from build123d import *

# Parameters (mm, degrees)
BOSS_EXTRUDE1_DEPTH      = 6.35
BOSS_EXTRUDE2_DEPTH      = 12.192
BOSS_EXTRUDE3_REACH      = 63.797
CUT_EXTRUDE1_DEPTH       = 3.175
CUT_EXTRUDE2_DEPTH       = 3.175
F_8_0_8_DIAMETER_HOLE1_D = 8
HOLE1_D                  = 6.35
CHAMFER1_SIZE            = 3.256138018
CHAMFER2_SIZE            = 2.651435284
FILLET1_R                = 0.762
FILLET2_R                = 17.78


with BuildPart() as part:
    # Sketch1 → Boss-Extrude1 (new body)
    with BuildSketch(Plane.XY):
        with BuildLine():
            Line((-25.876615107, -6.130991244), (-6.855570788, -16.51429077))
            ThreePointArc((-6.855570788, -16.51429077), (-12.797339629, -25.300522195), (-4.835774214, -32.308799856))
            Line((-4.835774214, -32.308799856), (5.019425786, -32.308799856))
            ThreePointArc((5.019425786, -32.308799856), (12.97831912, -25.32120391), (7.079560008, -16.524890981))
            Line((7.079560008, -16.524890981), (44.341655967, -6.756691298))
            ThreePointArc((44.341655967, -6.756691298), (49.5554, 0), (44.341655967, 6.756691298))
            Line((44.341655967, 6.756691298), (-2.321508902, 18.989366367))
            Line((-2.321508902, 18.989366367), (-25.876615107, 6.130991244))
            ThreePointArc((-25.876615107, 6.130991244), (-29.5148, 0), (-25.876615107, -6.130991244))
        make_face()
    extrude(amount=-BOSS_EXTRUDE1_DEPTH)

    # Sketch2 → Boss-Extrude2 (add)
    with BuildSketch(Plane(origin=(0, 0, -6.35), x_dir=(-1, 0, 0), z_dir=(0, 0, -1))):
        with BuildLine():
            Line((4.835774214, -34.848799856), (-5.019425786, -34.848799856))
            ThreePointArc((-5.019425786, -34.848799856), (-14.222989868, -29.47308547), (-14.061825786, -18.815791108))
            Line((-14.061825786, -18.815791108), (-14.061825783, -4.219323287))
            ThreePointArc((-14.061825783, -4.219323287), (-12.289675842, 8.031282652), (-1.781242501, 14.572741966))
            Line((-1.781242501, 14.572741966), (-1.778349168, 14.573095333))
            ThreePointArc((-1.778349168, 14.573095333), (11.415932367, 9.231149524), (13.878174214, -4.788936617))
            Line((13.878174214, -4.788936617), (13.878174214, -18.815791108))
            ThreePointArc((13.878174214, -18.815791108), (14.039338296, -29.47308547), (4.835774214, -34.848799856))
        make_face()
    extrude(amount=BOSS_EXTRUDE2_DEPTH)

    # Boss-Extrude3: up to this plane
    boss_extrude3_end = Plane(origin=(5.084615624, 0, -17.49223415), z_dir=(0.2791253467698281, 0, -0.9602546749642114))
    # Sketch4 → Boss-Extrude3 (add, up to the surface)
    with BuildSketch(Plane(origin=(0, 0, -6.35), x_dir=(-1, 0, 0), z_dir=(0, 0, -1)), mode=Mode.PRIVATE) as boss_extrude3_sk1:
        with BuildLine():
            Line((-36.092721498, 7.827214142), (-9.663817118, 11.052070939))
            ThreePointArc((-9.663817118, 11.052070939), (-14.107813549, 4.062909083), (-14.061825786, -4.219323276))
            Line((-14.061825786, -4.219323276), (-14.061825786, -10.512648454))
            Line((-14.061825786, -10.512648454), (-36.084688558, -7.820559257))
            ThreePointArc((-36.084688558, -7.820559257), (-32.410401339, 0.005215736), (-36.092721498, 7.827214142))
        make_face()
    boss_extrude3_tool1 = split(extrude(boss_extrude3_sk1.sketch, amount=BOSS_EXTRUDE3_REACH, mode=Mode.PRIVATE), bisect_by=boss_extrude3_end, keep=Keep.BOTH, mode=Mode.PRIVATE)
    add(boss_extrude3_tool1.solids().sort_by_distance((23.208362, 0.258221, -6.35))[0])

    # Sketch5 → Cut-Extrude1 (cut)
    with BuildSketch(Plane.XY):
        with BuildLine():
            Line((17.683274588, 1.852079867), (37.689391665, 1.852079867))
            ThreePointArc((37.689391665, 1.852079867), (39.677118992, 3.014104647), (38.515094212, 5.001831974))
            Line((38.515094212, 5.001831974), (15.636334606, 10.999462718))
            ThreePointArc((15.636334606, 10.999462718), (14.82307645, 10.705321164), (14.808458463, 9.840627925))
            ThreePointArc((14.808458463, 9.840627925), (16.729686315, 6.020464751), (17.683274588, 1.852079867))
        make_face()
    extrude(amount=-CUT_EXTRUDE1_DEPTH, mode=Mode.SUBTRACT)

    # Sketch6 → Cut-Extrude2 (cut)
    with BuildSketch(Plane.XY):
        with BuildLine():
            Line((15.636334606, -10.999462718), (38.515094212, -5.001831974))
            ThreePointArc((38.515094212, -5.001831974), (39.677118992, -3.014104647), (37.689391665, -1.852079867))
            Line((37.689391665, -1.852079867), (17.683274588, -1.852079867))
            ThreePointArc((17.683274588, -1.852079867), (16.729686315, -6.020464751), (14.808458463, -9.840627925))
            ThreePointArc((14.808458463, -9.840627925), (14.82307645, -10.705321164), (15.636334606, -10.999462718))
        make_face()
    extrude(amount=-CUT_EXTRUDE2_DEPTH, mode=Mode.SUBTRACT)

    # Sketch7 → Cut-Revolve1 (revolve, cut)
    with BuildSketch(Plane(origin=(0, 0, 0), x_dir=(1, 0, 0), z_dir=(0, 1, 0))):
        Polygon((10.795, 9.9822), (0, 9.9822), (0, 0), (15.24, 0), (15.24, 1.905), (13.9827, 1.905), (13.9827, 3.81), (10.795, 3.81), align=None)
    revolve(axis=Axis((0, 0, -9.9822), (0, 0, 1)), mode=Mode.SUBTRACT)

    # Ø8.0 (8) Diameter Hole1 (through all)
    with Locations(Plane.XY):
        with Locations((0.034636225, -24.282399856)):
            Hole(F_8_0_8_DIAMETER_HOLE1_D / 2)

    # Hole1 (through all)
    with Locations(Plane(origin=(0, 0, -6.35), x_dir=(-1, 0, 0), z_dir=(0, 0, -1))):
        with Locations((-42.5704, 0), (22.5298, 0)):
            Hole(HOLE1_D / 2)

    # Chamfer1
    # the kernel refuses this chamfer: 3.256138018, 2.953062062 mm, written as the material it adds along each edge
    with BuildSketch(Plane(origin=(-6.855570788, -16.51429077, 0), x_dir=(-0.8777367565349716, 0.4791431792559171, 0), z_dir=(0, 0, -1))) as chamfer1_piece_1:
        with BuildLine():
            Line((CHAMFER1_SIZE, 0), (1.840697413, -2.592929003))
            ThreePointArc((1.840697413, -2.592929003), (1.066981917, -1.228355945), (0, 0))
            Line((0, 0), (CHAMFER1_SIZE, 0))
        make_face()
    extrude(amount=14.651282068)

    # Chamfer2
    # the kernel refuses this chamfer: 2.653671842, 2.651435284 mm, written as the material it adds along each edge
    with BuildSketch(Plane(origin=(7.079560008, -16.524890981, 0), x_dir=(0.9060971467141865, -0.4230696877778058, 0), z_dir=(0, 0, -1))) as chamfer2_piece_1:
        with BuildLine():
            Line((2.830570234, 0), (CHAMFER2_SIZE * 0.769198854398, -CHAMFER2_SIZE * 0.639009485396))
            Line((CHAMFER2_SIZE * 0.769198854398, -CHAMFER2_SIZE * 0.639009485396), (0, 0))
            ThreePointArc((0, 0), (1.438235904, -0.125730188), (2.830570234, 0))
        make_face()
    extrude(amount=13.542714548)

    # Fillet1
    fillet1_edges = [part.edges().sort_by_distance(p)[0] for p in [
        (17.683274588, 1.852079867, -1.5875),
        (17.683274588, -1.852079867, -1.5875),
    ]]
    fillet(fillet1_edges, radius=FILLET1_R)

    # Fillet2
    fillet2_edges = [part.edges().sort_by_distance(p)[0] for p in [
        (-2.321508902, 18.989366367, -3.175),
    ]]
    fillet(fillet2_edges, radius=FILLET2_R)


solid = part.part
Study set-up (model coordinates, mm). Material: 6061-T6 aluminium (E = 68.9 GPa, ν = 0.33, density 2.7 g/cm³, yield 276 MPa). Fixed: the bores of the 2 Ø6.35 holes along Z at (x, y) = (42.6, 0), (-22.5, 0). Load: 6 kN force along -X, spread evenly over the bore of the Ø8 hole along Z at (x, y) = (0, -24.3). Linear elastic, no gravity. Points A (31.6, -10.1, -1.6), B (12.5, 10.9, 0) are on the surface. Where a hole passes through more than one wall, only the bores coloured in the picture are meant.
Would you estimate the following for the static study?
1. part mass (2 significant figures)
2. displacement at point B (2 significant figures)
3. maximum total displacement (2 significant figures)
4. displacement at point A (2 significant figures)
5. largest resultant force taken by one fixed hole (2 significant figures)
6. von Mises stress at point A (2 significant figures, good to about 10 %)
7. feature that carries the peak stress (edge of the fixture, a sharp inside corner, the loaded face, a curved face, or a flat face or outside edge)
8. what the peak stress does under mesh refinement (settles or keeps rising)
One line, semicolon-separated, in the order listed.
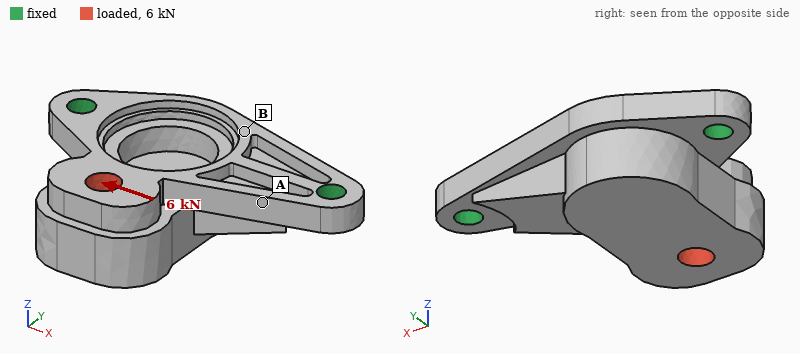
68 g; 31 µm; 82 µm; 19 µm; 4.0 kN; 67 MPa; a sharp inside corner; keeps rising
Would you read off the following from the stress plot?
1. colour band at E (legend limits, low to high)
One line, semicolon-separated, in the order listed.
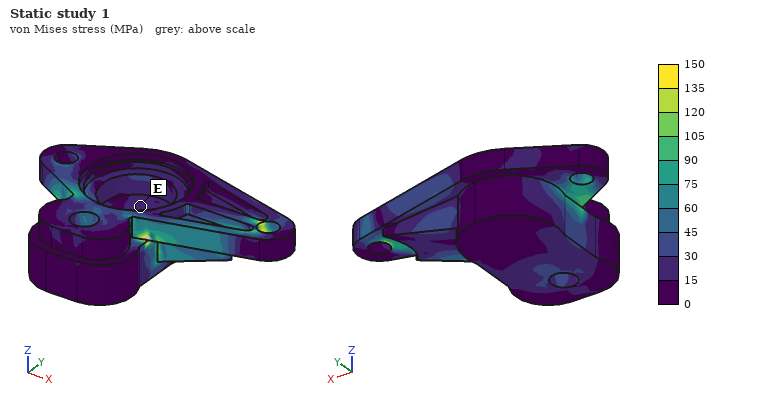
15 to 30 MPa
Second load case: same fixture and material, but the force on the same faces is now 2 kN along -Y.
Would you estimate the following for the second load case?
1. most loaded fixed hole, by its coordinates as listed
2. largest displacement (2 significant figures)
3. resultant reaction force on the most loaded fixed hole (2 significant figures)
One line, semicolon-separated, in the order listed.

(-22.5, 0); 69 µm; 1.3 kN
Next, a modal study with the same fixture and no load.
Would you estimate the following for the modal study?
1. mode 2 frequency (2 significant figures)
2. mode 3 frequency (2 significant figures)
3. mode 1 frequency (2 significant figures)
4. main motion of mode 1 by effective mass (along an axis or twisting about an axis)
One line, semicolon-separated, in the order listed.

7500 Hz; 9000 Hz; 2600 Hz; along Z
